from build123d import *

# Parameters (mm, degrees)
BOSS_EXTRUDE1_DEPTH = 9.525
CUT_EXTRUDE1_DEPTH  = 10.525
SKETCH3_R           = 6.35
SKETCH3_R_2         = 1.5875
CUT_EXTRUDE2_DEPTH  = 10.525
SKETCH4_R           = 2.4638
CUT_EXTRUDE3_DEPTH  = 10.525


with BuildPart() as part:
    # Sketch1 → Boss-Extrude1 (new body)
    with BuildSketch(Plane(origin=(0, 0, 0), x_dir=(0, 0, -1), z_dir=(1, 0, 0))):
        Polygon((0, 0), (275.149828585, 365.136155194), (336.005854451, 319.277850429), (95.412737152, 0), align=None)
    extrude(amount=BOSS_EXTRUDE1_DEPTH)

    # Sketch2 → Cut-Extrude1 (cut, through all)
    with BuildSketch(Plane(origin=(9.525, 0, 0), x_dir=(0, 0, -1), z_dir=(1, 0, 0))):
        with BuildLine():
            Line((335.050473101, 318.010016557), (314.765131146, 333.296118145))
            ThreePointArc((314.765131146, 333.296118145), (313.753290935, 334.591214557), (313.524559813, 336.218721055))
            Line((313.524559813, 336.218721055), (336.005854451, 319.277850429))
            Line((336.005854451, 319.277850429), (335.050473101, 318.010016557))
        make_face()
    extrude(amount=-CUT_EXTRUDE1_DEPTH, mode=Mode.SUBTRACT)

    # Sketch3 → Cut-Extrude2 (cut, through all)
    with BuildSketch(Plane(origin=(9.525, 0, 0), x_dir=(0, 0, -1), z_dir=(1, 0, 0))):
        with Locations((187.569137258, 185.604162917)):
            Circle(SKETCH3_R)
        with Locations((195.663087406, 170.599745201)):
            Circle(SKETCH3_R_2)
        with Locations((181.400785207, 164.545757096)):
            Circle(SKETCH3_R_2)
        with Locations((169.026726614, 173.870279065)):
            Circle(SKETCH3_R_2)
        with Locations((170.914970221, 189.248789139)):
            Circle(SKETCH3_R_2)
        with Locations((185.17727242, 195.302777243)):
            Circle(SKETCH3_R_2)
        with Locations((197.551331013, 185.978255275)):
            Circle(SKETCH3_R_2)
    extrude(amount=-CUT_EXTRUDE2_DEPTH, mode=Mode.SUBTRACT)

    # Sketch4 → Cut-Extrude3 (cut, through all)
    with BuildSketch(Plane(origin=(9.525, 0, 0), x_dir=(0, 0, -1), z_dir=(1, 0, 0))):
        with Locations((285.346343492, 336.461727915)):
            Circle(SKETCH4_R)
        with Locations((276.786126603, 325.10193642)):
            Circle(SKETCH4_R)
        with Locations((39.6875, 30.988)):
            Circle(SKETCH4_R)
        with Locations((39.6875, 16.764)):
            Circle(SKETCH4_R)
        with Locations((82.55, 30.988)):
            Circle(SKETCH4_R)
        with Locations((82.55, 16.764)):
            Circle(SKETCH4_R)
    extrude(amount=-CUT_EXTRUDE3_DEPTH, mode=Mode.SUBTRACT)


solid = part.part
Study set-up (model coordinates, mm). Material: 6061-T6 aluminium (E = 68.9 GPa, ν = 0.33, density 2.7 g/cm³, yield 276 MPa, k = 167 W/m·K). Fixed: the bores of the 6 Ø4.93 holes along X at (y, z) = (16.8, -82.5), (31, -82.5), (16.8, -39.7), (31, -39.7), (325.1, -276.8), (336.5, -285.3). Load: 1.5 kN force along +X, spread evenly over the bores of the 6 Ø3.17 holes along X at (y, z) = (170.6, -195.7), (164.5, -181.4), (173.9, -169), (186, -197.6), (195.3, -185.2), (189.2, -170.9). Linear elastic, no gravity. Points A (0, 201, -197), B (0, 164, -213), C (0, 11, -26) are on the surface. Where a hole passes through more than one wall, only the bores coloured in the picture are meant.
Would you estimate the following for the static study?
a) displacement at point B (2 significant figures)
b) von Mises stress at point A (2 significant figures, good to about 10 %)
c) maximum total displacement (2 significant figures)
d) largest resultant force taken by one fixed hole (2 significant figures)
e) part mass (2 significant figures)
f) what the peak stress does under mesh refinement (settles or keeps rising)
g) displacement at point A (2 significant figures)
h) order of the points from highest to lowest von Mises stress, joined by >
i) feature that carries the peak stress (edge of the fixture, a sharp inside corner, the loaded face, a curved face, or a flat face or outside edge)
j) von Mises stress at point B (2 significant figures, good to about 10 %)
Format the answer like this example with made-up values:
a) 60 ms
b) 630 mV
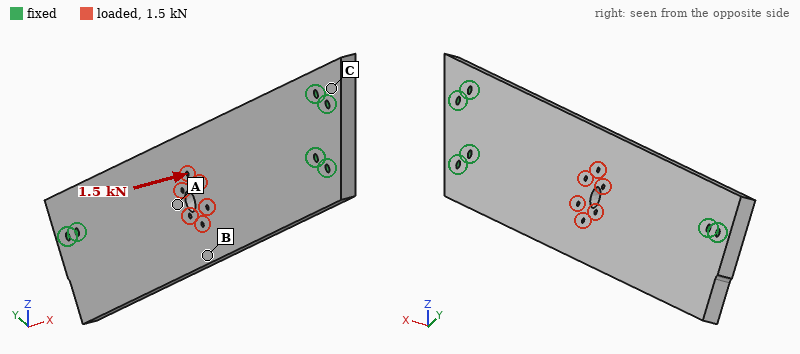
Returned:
a) 1.0 mm
b) 32 MPa
c) 1.0 mm
d) 2.7 kN
e) 830 g
f) keeps rising
g) 0.94 mm
h) B > A > C
i) edge of the fixture
j) 57 MPa
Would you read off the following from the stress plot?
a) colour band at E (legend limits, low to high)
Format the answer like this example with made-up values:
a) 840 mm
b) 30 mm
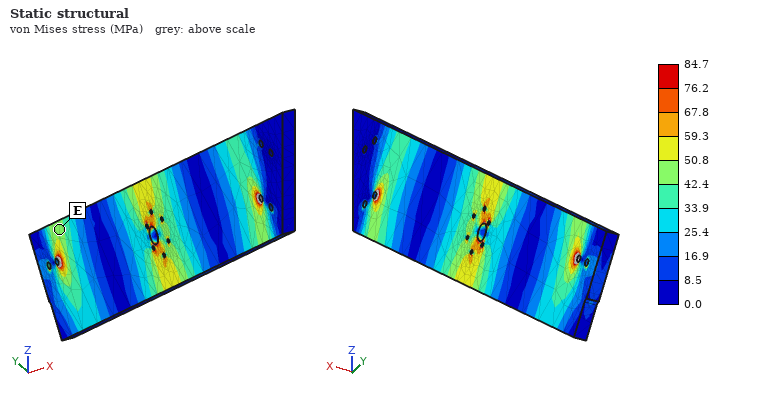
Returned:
a) 42.4 to 50.8 MPa
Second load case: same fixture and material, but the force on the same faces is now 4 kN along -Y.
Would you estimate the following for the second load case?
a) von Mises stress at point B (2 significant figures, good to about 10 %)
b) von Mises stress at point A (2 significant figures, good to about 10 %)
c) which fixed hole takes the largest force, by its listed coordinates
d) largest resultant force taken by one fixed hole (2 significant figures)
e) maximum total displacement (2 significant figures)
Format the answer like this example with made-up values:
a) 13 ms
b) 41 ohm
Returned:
a) 13 MPa
b) 4.6 MPa
c) (325.1, -276.8)
d) 3.0 kN
e) 54 µm
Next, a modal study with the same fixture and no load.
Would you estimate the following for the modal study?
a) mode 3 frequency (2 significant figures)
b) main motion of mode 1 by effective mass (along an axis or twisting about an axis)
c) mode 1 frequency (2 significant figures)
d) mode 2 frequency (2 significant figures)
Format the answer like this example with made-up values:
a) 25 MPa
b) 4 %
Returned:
a) 1100 Hz
b) along X
c) 370 Hz
d) 960 Hz
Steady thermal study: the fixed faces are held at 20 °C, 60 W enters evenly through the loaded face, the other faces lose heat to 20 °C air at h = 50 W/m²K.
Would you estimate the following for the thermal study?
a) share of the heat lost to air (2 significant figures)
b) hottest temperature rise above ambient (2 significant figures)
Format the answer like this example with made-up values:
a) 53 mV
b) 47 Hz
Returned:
a) 61 %
b) 27 K
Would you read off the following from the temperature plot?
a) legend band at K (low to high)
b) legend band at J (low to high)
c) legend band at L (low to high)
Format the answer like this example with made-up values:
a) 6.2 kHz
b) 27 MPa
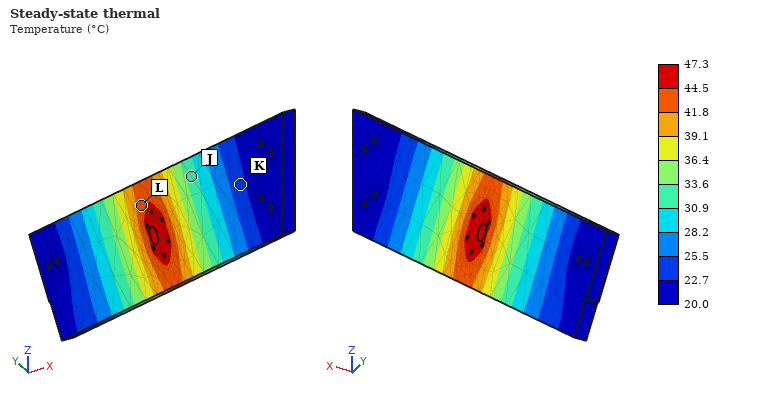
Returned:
a) 22.7 to 25.5 °C
b) 30.9 to 33.6 °C
c) 41.8 to 44.5 °C
